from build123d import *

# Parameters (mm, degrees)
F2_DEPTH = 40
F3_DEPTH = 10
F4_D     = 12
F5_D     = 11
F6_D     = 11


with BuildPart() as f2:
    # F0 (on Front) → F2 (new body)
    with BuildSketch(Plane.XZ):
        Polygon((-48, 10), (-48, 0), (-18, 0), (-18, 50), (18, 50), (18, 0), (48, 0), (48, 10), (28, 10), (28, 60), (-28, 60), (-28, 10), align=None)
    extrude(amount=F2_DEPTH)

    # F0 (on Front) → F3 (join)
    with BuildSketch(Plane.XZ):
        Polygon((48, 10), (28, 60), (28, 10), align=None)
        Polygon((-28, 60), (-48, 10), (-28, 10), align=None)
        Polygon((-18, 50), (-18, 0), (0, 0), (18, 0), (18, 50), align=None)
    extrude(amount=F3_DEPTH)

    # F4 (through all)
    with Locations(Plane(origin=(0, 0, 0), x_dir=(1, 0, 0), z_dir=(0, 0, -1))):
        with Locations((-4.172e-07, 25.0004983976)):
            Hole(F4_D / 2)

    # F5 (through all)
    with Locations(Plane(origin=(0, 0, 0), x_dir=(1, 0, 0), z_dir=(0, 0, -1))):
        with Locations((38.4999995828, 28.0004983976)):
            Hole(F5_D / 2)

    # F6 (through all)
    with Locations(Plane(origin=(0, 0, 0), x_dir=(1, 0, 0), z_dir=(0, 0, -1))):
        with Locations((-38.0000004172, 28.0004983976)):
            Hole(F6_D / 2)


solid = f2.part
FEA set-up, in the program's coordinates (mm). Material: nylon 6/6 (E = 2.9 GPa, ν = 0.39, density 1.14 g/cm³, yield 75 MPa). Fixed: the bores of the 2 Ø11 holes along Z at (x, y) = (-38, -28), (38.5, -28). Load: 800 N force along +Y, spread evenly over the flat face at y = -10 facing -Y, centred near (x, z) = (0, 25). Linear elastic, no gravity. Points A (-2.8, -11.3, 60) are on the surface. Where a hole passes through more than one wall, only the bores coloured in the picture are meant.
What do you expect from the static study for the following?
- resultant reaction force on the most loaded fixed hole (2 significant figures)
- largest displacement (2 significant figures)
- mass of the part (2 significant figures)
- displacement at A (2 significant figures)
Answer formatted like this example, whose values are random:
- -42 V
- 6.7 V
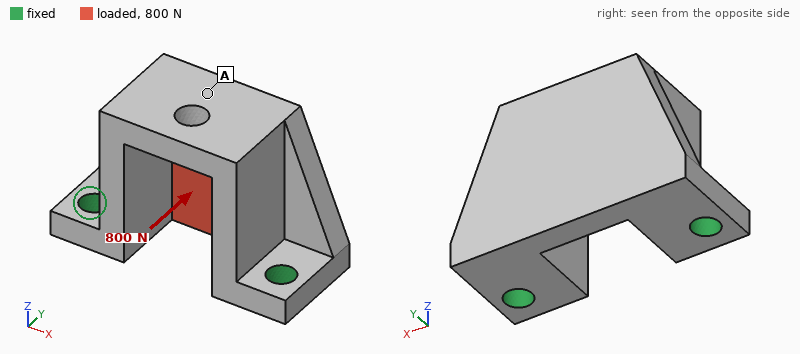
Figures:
- 450 N
- 0.41 mm
- 120 g
- 0.39 mm
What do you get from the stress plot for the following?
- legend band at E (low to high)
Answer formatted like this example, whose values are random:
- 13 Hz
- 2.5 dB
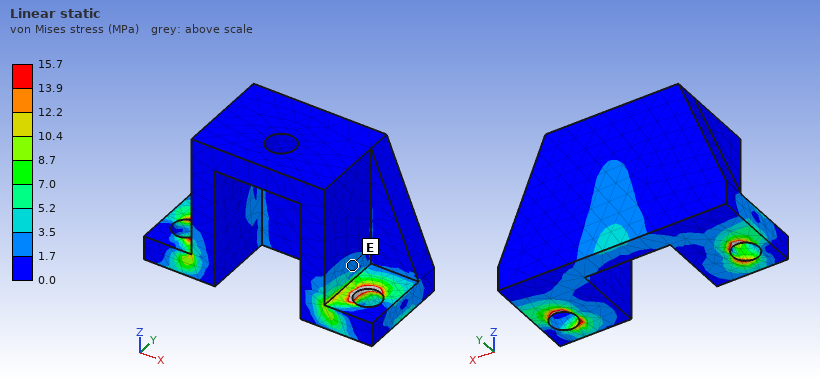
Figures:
- 1.7 to 3.5 MPa
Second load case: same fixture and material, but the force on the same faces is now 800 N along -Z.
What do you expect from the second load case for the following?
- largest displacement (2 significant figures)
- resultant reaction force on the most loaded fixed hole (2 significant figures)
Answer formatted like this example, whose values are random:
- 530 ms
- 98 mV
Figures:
- 0.30 mm
- 410 N
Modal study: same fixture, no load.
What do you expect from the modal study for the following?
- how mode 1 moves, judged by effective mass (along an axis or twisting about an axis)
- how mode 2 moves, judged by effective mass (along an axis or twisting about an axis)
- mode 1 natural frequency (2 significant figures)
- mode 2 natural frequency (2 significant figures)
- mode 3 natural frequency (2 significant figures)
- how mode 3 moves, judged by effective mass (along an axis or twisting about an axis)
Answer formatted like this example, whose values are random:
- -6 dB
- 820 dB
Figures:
- along Y
- along X
- 680 Hz
- 1100 Hz
- 2300 Hz
- along X
